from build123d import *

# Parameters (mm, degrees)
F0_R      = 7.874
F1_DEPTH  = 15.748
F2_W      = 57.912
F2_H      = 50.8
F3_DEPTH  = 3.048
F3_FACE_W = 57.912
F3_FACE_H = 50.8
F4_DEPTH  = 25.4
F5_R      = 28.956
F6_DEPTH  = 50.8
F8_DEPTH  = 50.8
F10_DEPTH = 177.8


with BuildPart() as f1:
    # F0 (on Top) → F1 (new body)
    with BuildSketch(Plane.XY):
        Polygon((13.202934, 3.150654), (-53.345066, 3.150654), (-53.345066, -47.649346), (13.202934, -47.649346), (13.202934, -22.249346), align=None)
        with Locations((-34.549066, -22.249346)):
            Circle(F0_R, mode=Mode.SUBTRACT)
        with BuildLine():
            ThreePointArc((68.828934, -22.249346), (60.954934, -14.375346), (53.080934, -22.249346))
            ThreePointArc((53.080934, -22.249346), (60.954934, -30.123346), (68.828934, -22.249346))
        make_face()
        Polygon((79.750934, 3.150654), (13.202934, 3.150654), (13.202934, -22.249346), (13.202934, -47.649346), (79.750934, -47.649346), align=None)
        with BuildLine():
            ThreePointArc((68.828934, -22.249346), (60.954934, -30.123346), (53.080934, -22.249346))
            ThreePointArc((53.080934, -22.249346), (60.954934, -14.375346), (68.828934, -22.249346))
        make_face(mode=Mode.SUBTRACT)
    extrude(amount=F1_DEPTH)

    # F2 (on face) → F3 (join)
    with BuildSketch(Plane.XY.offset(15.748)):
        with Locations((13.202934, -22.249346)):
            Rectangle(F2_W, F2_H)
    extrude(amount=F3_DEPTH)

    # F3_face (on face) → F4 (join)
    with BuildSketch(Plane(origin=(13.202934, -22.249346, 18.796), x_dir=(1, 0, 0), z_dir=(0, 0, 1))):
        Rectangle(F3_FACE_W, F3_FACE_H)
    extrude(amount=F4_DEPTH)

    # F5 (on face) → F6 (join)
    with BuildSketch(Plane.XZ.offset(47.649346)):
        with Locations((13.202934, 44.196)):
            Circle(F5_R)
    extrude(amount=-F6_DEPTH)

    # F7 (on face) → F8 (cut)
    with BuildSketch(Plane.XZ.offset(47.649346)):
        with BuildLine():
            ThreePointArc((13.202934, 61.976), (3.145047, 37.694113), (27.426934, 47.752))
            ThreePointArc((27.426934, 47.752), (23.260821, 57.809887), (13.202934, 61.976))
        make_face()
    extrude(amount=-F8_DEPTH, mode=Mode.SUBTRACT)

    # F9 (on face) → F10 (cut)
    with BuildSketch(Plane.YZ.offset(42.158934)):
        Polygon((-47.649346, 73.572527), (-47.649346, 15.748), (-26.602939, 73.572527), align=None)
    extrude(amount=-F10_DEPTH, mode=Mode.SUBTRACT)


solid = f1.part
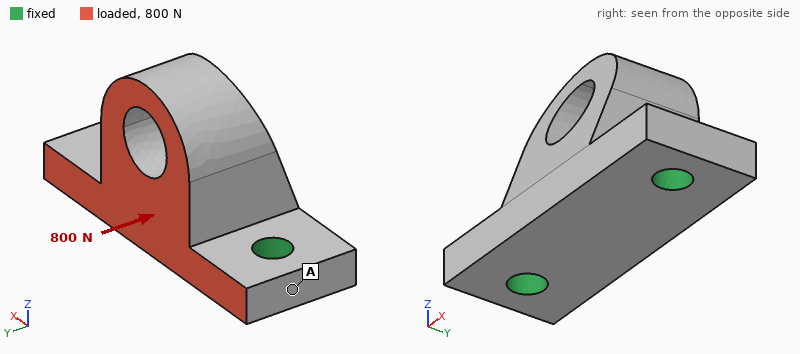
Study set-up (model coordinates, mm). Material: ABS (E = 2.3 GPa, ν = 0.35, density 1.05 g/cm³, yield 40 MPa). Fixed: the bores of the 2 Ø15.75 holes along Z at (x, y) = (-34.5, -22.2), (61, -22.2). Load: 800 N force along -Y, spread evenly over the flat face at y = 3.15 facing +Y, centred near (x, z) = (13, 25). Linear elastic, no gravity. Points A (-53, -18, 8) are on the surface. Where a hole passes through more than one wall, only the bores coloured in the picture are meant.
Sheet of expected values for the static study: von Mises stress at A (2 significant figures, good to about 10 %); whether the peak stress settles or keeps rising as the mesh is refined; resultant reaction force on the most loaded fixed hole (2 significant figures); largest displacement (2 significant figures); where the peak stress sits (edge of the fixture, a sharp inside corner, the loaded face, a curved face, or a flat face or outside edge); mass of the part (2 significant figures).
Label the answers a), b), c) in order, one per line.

a) 0.62 MPa
b) keeps rising
c) 400 N
d) 0.20 mm
e) edge of the fixture
f) 210 g
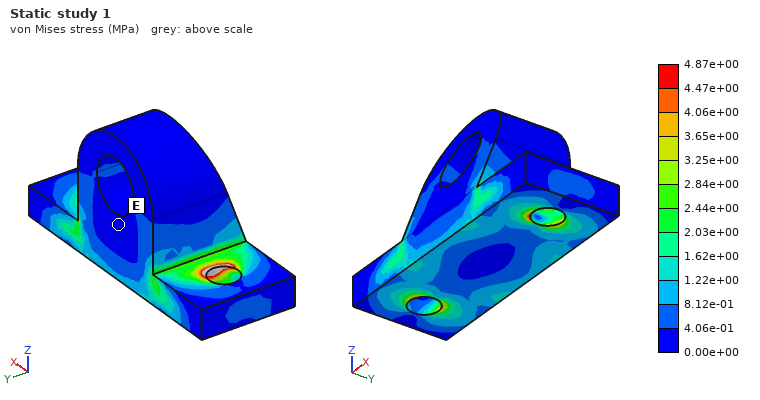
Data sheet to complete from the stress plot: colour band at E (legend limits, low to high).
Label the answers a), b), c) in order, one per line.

a) 0.00e+00 to 4.06e-01 MPa
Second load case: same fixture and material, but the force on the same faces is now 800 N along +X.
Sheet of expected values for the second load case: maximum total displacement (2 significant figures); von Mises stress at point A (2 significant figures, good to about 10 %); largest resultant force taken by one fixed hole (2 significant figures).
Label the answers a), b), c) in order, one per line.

a) 61 µm
b) 0.55 MPa
c) 480 N
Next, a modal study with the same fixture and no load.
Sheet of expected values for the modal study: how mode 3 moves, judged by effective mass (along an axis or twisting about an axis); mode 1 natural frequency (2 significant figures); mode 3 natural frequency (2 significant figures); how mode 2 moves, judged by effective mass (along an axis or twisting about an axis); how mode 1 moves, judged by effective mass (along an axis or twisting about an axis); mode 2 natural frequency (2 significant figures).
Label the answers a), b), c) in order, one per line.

a) along Z
b) 930 Hz
c) 2100 Hz
d) along X
e) along Y
f) 1900 Hz
